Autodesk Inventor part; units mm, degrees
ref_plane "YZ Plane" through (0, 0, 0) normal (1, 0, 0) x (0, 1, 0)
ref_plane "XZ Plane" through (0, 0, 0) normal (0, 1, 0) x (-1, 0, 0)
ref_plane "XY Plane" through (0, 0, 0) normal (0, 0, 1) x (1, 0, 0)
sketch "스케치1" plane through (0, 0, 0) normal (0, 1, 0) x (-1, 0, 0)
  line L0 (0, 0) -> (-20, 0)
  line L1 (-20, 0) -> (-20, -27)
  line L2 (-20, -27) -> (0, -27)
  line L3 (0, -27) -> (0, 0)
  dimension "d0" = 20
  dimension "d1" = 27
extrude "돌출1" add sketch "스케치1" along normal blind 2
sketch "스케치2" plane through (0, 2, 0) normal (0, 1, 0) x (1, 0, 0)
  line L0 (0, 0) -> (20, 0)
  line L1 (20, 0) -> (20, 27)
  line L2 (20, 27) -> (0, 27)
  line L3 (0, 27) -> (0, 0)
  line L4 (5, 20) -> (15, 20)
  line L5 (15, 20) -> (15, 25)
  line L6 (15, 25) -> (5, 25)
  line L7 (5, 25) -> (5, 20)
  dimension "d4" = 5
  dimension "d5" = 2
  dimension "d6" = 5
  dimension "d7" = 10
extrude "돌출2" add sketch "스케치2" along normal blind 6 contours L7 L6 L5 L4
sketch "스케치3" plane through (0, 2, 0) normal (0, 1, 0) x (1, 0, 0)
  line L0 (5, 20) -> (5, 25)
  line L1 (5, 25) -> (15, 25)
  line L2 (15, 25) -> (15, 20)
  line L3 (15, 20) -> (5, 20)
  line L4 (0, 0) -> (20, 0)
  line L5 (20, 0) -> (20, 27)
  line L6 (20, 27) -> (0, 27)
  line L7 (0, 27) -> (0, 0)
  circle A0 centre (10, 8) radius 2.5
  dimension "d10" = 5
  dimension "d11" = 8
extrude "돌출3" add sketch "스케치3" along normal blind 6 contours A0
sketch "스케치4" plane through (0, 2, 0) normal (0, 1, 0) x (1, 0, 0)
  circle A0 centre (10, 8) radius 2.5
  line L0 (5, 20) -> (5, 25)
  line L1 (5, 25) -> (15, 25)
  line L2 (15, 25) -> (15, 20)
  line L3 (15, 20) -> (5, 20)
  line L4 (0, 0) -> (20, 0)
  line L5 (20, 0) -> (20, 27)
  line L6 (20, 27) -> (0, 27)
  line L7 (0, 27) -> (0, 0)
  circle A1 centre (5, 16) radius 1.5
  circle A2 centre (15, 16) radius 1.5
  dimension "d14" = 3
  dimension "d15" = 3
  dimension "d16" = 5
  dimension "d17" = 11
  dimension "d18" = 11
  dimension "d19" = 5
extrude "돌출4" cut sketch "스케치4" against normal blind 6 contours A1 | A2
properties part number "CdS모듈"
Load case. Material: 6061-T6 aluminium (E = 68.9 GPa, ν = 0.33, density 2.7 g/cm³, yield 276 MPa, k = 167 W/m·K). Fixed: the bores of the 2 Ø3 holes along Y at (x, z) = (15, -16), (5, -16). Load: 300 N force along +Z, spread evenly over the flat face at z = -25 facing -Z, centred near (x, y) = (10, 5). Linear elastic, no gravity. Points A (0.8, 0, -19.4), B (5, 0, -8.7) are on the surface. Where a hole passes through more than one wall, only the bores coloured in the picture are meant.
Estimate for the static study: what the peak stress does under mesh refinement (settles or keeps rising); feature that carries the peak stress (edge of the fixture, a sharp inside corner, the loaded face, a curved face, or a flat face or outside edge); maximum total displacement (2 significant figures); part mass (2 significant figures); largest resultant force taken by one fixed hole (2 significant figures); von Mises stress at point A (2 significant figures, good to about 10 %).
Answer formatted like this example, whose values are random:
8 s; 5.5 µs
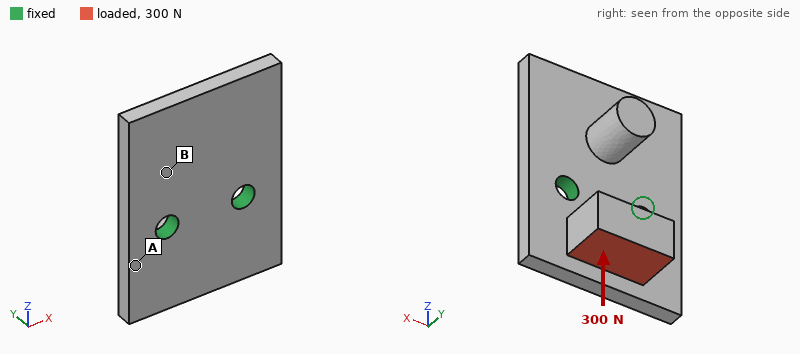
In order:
keeps rising; edge of the fixture; 58 µm; 4.0 g; 160 N; 57 MPa
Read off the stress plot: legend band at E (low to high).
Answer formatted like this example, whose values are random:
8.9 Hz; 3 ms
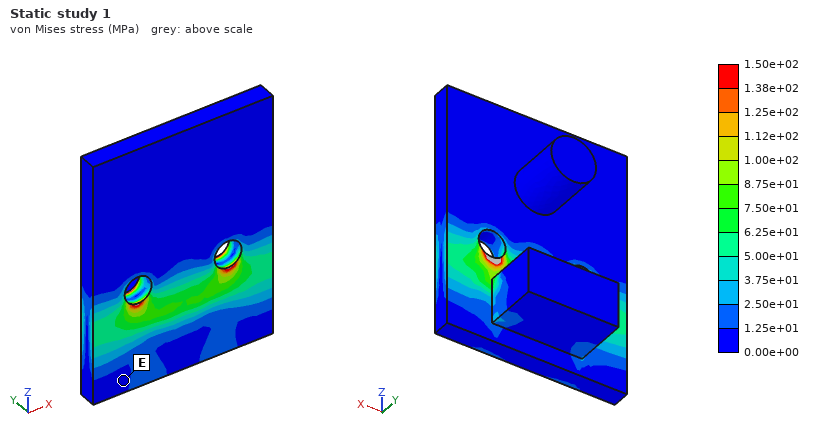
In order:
0.00e+00 to 1.25e+01 MPa
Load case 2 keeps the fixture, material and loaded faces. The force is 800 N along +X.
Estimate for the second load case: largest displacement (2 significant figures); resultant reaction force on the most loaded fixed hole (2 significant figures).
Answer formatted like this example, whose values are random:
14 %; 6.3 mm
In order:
31 µm; 770 N
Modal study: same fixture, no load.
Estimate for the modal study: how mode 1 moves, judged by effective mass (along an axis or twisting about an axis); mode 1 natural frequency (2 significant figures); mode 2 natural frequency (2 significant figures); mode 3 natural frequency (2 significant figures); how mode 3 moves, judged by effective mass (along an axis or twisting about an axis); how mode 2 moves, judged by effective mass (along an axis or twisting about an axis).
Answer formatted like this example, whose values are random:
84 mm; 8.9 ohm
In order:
along Y; 6600 Hz; 10 kHz; 13 kHz; twisting about Z; along Y
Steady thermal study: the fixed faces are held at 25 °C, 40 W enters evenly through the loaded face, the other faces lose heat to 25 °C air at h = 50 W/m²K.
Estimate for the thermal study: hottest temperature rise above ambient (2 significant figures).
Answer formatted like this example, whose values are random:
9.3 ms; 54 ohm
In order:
59 K
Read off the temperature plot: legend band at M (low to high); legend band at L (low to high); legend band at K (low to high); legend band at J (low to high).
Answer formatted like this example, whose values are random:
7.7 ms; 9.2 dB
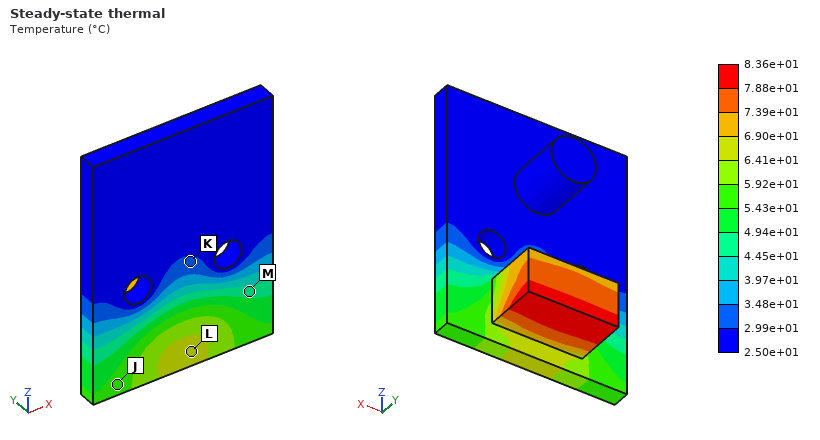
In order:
4.45e+01 to 4.94e+01 °C; 6.41e+01 to 6.90e+01 °C; 2.99e+01 to 3.48e+01 °C; 5.43e+01 to 5.92e+01 °C
